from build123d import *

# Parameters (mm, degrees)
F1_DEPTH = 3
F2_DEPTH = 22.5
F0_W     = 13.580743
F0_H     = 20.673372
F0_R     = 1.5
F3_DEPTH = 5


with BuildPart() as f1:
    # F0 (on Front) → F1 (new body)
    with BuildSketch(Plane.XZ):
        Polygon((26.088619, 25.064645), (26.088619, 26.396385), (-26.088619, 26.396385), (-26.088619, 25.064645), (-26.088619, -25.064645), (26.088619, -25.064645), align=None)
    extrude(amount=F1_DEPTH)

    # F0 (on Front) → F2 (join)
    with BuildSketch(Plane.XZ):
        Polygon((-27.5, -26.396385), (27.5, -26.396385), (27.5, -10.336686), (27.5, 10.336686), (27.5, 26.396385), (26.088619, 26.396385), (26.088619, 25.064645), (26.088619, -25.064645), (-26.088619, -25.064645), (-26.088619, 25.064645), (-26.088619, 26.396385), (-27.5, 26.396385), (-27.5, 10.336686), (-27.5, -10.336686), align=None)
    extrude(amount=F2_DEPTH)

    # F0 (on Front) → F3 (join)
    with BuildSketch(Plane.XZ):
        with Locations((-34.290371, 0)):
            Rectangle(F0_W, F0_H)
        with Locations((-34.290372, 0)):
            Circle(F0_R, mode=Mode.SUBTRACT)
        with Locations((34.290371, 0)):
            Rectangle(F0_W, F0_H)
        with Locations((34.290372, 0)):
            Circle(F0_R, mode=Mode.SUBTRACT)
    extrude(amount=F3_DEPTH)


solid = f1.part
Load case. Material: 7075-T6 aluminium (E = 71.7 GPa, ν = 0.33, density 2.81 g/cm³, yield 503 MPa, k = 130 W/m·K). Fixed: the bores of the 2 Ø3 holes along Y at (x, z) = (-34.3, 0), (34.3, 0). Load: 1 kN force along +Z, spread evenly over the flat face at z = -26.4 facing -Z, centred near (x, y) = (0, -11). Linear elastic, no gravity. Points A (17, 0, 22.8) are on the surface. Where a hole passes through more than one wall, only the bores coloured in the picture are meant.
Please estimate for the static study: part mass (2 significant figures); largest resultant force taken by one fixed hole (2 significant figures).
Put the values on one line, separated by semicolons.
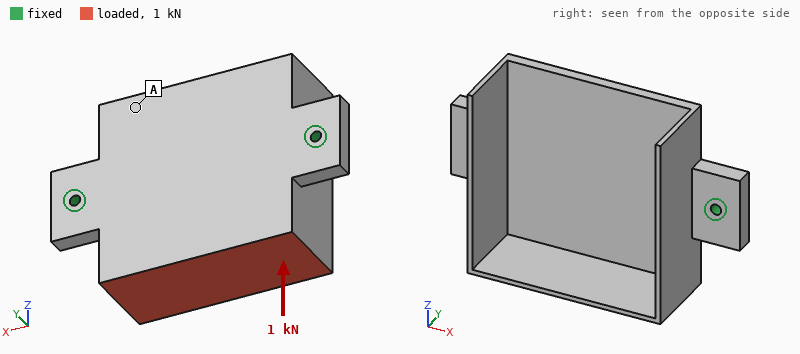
44 g; 500 N
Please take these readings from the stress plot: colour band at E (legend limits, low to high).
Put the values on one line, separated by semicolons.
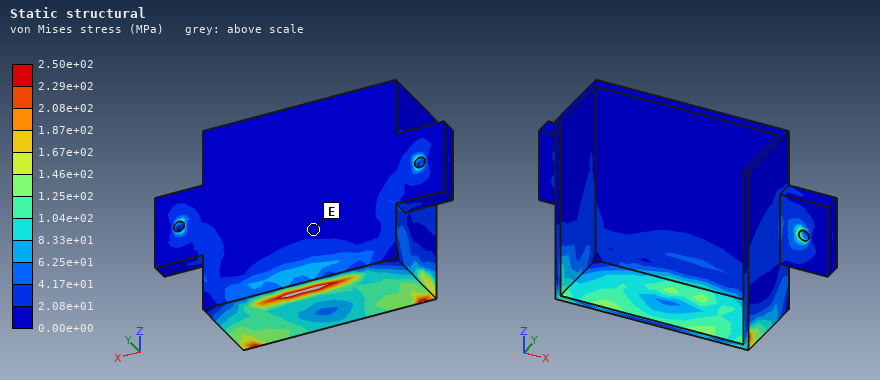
0.00e+00 to 2.08e+01 MPa
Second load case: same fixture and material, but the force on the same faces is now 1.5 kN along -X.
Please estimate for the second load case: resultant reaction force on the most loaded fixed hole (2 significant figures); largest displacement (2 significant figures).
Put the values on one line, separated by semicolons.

980 N; 0.13 mm
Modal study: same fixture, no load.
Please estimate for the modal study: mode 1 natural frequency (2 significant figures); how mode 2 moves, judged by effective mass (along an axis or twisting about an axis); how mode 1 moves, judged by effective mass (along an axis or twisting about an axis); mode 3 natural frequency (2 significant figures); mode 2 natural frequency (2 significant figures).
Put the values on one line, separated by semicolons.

2600 Hz; along Y; twisting about X; 3500 Hz; 3200 Hz
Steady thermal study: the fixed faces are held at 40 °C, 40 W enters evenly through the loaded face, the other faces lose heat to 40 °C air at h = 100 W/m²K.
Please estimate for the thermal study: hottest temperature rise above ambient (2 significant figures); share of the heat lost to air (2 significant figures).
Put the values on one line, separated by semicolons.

58 K; 51 %
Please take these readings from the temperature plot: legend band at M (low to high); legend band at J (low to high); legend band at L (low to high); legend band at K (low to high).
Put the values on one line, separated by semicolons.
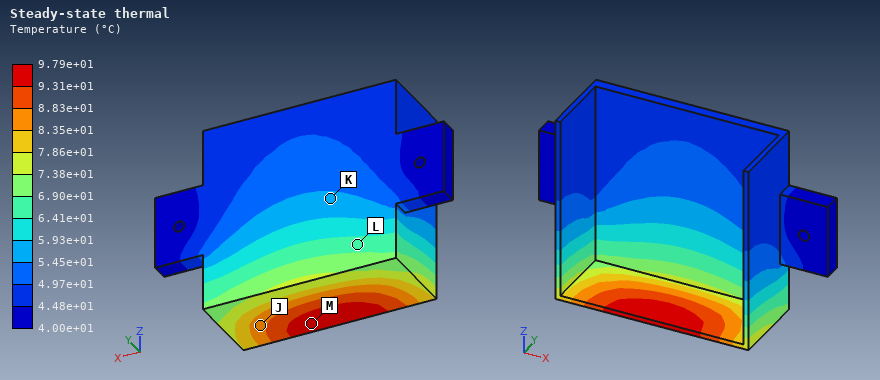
9.31e+01 to 9.79e+01 °C; 8.35e+01 to 8.83e+01 °C; 6.41e+01 to 6.90e+01 °C; 5.45e+01 to 5.93e+01 °C
